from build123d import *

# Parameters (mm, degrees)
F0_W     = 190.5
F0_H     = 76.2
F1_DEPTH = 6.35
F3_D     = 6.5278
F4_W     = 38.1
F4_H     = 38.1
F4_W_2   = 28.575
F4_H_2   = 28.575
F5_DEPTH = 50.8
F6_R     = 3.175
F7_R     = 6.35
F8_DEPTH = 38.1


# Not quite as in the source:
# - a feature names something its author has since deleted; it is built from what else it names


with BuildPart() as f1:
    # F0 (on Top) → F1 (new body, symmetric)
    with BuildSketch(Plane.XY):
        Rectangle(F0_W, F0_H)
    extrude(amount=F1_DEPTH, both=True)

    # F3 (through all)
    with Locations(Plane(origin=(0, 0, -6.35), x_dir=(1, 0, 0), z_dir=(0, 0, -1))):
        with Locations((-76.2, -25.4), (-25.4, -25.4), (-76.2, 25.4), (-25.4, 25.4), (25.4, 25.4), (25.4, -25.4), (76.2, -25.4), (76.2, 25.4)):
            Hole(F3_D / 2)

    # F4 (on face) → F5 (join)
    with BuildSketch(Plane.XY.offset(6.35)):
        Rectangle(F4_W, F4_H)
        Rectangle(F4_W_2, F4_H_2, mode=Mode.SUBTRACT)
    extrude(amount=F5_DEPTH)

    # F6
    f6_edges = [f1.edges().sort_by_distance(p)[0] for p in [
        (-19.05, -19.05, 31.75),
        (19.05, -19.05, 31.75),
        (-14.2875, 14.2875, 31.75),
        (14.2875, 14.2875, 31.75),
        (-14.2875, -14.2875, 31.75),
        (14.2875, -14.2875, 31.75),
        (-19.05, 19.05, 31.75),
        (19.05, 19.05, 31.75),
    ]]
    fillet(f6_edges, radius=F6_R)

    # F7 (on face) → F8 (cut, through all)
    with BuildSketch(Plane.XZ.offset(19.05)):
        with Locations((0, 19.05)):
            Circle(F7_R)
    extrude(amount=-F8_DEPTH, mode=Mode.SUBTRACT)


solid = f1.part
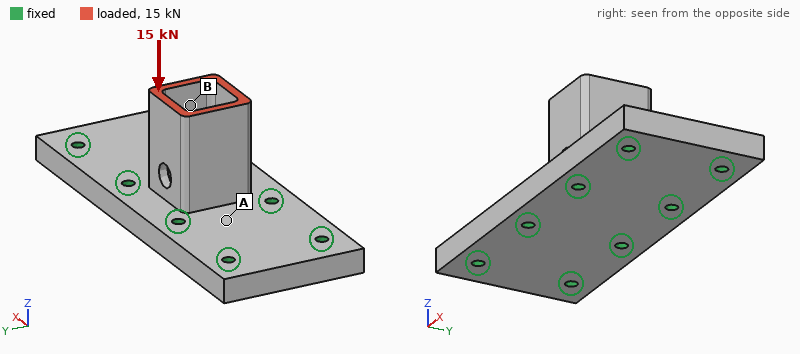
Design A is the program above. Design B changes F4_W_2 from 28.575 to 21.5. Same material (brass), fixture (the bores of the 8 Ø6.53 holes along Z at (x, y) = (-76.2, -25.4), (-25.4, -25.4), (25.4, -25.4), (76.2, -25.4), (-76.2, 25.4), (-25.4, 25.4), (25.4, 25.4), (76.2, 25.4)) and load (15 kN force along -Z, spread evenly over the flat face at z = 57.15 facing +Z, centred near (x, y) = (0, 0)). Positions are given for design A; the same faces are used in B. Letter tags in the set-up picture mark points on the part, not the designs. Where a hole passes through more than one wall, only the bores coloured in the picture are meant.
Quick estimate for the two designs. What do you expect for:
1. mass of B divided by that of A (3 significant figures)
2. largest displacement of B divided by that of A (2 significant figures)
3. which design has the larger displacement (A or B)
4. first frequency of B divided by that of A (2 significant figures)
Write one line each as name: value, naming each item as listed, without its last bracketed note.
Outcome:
mass of B divided by that of A: 1.05
largest displacement of B divided by that of A: 0.85
which design has the larger displacement: A
first frequency of B divided by that of A: 0.93
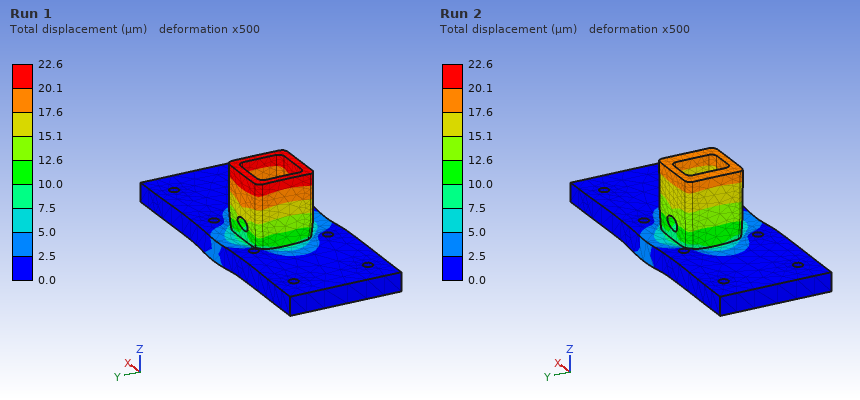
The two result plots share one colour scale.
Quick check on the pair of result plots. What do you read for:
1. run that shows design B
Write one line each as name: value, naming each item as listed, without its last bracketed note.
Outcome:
run that shows design B: Run 2
